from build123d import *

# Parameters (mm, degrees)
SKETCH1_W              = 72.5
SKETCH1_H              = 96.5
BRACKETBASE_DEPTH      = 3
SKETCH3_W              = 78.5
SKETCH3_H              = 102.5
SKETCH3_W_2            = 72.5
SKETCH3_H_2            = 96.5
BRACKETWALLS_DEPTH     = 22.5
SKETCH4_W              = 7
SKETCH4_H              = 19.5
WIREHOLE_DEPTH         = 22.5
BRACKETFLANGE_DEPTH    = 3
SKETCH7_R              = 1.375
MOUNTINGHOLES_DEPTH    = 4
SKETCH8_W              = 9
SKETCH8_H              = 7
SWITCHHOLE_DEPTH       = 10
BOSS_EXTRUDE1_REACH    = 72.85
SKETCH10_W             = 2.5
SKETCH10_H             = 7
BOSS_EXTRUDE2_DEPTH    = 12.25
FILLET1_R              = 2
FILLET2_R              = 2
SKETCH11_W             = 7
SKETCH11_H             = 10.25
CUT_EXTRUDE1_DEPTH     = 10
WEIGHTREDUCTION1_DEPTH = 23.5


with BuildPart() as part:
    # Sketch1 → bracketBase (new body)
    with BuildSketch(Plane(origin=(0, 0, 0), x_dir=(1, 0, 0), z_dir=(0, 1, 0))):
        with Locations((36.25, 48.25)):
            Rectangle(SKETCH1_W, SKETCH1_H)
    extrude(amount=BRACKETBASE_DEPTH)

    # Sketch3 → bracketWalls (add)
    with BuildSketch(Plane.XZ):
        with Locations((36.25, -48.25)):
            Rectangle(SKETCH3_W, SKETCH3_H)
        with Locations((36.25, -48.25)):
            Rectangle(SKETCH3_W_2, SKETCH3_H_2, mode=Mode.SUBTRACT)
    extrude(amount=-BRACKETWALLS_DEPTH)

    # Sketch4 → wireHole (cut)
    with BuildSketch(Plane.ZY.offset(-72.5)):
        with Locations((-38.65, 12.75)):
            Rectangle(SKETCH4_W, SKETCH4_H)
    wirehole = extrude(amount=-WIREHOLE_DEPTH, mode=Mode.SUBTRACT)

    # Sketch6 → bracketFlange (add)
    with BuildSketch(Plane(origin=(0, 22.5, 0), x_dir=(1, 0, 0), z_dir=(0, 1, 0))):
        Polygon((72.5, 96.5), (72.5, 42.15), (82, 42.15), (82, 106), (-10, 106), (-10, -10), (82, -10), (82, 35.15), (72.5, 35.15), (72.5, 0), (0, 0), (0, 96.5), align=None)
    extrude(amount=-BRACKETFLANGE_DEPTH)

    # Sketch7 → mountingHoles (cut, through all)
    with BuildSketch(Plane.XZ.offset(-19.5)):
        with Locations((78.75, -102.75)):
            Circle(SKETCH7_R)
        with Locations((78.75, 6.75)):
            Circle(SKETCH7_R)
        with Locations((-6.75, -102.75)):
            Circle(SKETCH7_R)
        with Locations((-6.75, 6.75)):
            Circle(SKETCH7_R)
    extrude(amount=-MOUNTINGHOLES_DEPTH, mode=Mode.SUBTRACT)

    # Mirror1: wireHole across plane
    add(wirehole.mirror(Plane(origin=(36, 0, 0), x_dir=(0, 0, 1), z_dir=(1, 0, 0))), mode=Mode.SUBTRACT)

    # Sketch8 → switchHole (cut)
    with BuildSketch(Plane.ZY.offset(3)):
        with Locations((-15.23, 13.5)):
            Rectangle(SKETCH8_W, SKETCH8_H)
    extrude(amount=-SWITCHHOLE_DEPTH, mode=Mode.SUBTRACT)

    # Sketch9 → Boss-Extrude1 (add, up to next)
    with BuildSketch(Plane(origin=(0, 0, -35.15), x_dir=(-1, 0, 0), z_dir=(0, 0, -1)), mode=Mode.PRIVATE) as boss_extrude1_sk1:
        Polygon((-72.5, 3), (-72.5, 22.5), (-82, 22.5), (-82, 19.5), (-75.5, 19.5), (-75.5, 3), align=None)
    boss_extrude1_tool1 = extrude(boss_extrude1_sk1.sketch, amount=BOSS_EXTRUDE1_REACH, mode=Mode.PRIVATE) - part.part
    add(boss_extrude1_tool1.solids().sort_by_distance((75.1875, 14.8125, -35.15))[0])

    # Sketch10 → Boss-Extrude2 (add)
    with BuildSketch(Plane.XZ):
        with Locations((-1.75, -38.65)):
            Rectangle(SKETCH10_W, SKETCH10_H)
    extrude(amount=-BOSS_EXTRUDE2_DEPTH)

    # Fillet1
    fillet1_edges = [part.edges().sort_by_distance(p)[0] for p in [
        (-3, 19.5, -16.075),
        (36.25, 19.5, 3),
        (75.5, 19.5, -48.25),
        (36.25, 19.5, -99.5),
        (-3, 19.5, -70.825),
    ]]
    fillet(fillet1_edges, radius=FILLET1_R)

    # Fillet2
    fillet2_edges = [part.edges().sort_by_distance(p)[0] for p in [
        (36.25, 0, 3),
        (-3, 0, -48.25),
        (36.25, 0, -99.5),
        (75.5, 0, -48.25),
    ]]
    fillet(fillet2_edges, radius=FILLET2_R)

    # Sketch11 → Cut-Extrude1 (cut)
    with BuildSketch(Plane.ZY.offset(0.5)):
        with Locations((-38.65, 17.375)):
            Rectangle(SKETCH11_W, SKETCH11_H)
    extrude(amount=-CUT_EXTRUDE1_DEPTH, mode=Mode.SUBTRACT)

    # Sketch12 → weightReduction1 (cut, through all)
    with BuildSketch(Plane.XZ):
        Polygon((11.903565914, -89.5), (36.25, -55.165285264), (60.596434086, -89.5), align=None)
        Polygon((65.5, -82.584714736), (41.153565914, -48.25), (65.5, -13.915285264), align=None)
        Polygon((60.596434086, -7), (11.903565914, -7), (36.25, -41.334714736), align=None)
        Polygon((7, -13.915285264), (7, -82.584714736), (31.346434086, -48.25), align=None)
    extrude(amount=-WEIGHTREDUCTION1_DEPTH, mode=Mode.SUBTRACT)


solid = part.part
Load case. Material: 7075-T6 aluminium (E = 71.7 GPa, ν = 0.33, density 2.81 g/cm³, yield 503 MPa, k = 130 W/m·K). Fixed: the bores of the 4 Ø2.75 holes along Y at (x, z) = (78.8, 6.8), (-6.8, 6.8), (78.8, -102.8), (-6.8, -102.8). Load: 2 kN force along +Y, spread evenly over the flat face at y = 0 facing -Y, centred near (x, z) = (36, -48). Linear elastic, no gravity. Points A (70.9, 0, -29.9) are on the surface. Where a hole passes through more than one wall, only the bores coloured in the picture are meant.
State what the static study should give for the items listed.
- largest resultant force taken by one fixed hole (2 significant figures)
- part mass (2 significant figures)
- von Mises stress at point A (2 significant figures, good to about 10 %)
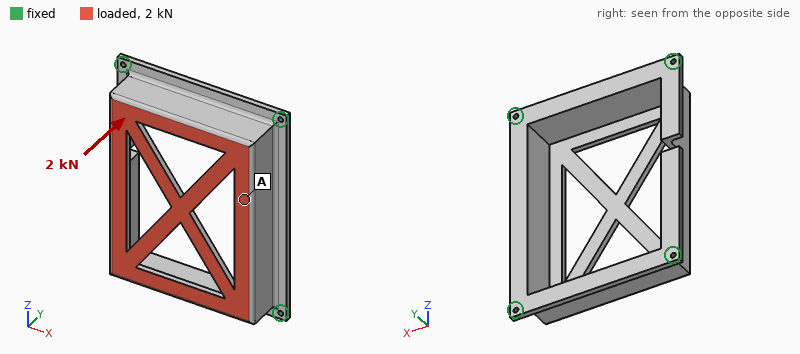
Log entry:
860 N
120 g
17 MPa
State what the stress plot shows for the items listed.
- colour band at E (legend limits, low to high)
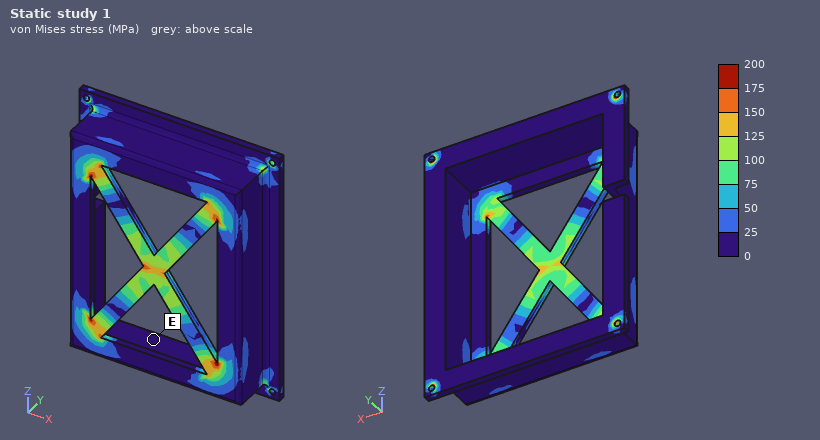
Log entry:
0 to 25 MPa
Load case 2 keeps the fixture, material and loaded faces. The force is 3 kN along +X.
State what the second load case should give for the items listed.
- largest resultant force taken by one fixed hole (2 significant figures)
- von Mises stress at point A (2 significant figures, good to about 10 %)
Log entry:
880 N
21 MPa
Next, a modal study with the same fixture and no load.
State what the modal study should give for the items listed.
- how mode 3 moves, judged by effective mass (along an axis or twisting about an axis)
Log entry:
along X
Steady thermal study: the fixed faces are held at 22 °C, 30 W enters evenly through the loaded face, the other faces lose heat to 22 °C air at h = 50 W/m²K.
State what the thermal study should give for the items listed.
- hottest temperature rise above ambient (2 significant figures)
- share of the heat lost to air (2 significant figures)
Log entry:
28 K
48 %
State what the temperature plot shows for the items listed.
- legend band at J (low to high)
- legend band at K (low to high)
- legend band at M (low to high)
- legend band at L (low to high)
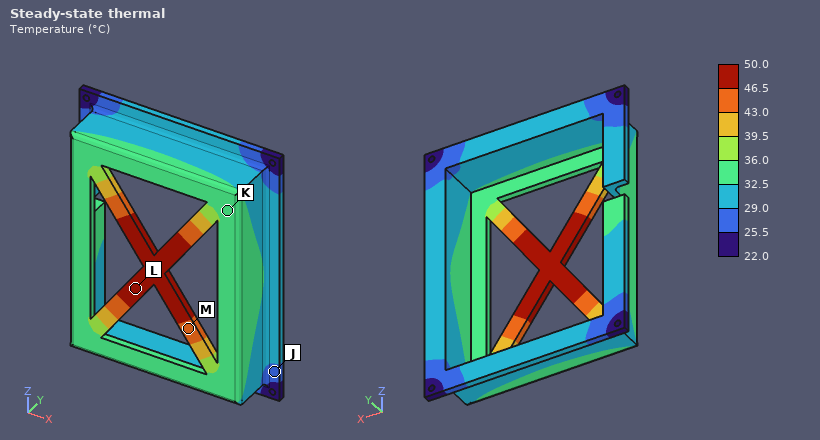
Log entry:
25.5 to 29.0 °C
32.5 to 36.0 °C
43.0 to 46.5 °C
46.5 to 50.0 °C
